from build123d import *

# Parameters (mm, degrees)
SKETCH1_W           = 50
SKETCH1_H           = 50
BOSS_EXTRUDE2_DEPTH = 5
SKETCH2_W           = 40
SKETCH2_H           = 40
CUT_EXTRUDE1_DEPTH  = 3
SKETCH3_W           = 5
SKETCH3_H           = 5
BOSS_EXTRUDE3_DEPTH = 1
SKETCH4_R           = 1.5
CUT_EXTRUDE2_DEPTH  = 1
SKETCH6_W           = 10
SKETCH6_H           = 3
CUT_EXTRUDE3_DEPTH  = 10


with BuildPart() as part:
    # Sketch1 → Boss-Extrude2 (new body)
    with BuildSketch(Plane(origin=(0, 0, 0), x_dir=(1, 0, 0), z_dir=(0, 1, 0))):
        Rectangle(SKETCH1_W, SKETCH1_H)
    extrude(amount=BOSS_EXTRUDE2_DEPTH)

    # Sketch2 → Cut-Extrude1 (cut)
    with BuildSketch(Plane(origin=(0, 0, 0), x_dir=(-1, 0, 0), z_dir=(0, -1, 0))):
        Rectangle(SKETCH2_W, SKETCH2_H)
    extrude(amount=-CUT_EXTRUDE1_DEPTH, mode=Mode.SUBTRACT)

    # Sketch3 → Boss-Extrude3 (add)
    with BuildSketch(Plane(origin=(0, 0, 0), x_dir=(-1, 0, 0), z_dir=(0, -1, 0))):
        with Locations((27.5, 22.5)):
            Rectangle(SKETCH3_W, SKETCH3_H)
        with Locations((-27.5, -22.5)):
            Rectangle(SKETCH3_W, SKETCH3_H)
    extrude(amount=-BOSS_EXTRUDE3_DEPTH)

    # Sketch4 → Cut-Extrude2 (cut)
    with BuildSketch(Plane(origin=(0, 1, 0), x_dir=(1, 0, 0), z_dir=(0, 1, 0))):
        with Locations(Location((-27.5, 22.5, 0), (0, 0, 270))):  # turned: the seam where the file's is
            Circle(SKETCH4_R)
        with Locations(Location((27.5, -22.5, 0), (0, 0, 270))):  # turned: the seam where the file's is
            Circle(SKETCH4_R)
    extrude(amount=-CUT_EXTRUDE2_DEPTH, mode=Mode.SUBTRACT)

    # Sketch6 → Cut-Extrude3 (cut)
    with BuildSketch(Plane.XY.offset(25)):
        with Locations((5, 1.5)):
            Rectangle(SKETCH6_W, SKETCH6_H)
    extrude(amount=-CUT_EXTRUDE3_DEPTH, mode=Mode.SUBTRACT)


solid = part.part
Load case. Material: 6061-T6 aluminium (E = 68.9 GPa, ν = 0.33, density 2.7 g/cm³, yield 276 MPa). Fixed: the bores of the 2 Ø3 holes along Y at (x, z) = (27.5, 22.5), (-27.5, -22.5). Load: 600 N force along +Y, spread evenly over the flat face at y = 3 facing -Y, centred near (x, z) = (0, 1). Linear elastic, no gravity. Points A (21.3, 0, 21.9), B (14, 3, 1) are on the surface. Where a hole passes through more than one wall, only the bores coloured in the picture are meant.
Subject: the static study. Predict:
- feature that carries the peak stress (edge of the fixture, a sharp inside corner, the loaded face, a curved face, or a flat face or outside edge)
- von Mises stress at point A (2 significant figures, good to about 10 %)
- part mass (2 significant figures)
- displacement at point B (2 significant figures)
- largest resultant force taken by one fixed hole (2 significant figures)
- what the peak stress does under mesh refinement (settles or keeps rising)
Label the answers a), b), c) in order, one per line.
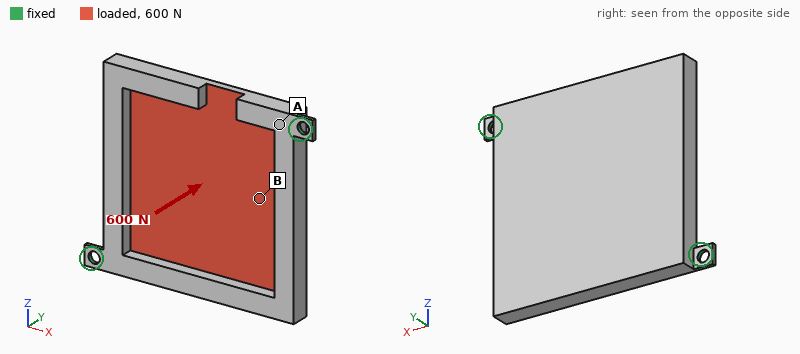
a) edge of the fixture
b) 66 MPa
c) 20 g
d) 0.15 mm
e) 1.2 kN
f) keeps rising
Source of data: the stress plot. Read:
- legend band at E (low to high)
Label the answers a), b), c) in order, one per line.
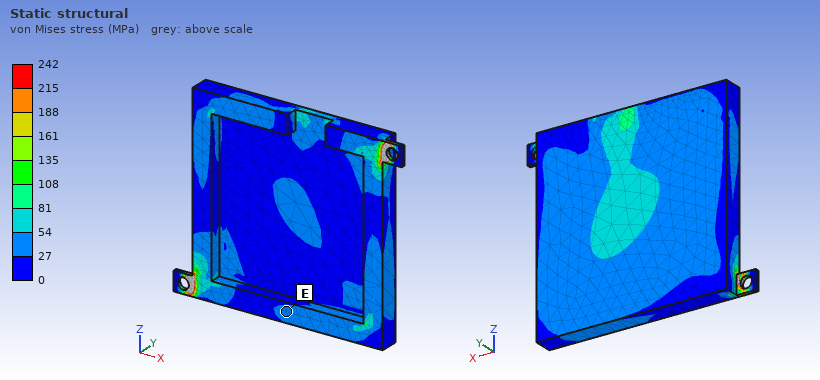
a) 27 to 54 MPa
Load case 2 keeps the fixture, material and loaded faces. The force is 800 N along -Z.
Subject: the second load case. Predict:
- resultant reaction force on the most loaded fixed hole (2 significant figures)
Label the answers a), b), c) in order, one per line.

a) 400 N
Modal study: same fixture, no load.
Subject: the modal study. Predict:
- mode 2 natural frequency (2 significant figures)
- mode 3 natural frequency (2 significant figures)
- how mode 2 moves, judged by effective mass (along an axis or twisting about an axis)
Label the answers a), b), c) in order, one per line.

a) 1900 Hz
b) 4000 Hz
c) along Y
